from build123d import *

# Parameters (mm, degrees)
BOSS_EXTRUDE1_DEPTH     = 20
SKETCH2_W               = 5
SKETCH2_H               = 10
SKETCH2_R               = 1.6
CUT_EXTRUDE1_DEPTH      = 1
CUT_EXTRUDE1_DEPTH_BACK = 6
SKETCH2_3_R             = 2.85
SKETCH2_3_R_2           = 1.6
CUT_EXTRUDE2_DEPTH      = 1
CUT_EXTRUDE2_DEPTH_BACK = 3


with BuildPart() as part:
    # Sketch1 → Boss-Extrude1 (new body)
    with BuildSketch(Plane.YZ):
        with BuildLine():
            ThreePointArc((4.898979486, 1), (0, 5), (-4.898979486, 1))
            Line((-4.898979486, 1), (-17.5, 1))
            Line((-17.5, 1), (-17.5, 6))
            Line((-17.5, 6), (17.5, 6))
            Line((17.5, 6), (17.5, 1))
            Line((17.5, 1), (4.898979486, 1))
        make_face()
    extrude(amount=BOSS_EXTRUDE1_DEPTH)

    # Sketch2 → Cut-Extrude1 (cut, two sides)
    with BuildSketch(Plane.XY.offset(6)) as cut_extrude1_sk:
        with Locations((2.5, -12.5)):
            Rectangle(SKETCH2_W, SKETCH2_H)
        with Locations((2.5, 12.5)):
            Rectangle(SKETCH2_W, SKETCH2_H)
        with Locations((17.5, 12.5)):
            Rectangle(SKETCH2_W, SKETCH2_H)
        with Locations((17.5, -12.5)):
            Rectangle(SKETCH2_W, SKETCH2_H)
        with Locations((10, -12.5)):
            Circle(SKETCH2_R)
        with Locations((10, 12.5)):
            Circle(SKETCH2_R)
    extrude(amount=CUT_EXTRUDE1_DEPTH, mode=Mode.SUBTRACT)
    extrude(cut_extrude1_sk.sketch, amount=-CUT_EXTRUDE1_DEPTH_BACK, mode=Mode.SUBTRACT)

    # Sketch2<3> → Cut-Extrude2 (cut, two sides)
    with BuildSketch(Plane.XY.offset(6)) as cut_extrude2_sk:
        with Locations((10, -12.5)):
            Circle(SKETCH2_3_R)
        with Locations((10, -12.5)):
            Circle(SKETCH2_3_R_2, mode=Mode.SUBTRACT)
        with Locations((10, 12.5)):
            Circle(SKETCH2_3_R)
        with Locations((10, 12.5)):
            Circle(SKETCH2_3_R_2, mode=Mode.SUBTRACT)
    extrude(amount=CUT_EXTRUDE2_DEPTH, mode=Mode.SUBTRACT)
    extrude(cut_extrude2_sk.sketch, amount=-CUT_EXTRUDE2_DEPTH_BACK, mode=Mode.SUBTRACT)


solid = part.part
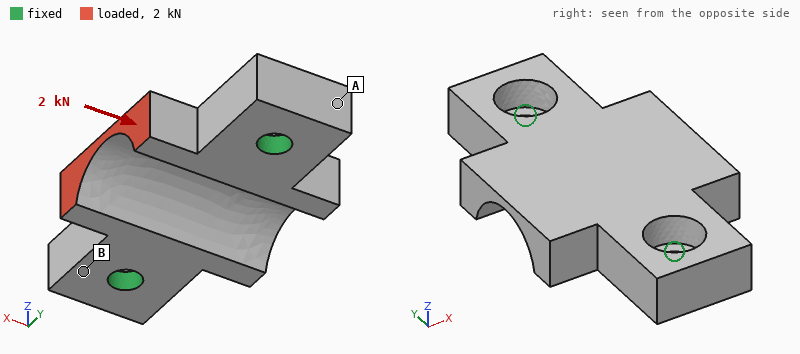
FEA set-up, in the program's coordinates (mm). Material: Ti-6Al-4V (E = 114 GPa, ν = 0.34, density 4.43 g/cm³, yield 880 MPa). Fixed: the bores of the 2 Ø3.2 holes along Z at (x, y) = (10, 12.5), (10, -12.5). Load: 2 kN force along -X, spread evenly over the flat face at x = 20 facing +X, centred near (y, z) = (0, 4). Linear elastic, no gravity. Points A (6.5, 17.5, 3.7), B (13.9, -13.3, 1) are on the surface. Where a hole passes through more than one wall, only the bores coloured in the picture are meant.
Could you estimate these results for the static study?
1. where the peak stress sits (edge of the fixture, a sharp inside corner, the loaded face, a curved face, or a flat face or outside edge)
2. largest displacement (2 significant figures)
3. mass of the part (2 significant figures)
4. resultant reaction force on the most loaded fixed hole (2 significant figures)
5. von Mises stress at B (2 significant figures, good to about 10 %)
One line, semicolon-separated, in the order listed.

edge of the fixture; 40 µm; 7.7 g; 1.0 kN; 59 MPa
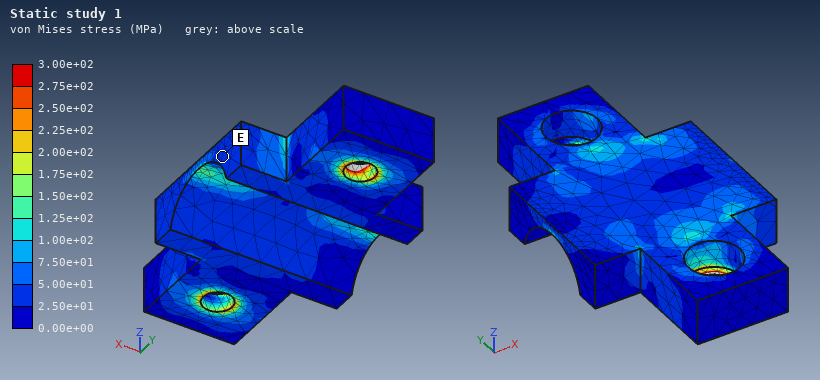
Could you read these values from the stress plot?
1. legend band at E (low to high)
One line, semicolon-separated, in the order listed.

2.50e+01 to 5.00e+01 MPa
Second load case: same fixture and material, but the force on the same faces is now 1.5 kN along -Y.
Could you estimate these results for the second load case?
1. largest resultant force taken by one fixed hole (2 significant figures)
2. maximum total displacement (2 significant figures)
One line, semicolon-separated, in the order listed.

940 N; 31 µm
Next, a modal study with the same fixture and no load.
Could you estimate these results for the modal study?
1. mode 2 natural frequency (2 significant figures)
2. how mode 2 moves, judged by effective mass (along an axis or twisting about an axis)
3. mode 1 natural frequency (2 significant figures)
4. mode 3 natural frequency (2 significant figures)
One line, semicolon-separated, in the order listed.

24 kHz; along Z; 15 kHz; 25 kHz
